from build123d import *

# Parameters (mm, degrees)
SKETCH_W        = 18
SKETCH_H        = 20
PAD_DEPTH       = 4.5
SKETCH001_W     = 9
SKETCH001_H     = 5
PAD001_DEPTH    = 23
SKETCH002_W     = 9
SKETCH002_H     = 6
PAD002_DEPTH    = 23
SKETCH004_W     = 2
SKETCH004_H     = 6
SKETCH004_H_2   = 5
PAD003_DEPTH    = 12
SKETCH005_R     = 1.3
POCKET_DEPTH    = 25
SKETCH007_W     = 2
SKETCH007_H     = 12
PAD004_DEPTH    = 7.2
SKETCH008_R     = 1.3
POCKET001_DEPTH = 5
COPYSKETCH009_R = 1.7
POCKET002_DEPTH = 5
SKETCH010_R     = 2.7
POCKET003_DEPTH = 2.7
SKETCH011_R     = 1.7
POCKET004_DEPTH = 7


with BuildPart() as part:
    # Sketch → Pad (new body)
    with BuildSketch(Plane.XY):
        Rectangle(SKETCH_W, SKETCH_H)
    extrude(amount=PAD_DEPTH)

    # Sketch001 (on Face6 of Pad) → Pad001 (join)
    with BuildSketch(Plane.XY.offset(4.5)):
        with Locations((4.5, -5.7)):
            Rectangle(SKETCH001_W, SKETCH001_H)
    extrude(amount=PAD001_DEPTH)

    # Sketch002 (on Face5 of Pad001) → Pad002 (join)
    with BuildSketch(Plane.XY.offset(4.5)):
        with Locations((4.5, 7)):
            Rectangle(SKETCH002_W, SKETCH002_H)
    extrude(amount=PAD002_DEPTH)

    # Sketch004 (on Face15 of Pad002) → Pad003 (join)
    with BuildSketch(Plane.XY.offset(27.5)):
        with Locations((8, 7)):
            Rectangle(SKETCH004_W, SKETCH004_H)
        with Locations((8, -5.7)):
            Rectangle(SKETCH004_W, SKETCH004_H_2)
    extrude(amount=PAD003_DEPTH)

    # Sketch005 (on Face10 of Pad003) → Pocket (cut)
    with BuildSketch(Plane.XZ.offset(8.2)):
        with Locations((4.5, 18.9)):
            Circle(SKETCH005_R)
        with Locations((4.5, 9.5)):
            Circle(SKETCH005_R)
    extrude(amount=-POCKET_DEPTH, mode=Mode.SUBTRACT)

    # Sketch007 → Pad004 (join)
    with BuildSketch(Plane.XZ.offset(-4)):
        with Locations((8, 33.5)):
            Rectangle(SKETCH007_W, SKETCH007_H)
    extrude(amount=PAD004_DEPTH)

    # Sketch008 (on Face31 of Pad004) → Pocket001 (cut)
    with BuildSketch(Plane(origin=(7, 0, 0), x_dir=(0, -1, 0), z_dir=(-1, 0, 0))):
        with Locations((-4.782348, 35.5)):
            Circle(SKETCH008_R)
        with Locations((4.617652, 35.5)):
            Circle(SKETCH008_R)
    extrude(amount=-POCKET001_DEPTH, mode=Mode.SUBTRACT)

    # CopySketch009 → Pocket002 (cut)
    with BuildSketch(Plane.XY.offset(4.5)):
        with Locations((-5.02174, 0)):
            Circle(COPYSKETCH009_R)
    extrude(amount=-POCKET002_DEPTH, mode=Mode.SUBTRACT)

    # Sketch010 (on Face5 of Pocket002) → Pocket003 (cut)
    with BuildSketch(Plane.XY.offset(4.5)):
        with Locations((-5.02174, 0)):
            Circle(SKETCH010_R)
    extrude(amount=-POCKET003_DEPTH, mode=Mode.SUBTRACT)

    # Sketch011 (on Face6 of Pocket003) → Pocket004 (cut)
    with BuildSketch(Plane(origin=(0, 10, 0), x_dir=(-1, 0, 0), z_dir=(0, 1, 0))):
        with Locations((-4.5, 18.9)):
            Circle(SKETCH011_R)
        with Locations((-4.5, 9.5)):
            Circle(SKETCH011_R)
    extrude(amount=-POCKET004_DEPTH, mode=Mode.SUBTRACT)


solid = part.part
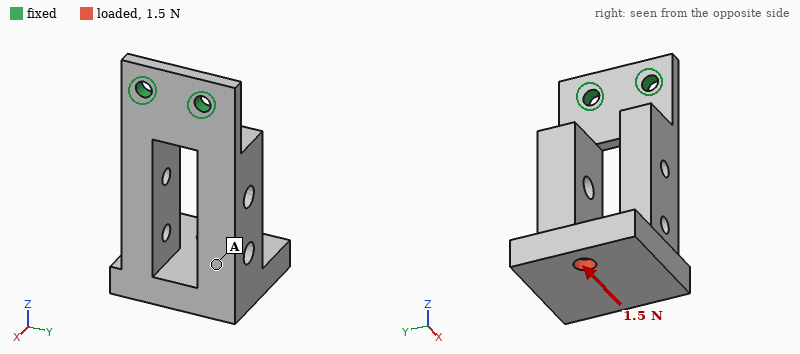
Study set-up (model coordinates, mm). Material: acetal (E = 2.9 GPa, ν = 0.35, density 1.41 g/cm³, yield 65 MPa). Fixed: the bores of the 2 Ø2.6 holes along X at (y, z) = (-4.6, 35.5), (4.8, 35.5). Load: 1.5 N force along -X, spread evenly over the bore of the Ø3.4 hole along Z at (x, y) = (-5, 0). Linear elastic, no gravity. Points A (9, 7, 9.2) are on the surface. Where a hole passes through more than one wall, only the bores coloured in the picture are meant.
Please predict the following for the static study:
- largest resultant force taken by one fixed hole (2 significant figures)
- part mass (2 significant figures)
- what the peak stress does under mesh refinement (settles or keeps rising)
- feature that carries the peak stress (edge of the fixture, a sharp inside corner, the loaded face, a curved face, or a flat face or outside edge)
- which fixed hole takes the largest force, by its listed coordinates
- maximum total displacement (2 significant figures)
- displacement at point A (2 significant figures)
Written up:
0.82 N
5.7 g
keeps rising
edge of the fixture
(4.8, 35.5)
0.44 mm
0.27 mm
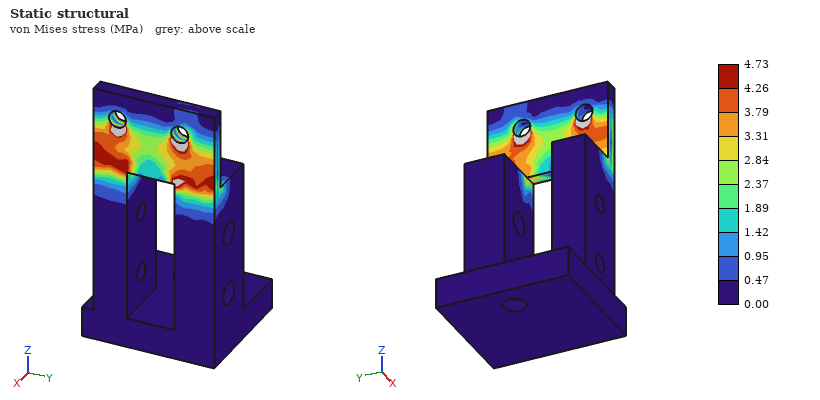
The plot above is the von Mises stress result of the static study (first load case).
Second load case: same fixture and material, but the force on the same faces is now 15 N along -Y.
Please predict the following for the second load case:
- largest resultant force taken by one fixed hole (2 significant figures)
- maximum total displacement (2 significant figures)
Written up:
48 N
0.47 mm
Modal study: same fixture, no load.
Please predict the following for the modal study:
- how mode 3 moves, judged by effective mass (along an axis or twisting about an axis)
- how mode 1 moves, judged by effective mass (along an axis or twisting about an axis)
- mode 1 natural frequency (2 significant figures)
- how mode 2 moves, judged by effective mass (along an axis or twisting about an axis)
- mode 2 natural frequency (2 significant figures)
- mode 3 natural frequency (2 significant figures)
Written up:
along Y
along X
180 Hz
along Y
690 Hz
1100 Hz
